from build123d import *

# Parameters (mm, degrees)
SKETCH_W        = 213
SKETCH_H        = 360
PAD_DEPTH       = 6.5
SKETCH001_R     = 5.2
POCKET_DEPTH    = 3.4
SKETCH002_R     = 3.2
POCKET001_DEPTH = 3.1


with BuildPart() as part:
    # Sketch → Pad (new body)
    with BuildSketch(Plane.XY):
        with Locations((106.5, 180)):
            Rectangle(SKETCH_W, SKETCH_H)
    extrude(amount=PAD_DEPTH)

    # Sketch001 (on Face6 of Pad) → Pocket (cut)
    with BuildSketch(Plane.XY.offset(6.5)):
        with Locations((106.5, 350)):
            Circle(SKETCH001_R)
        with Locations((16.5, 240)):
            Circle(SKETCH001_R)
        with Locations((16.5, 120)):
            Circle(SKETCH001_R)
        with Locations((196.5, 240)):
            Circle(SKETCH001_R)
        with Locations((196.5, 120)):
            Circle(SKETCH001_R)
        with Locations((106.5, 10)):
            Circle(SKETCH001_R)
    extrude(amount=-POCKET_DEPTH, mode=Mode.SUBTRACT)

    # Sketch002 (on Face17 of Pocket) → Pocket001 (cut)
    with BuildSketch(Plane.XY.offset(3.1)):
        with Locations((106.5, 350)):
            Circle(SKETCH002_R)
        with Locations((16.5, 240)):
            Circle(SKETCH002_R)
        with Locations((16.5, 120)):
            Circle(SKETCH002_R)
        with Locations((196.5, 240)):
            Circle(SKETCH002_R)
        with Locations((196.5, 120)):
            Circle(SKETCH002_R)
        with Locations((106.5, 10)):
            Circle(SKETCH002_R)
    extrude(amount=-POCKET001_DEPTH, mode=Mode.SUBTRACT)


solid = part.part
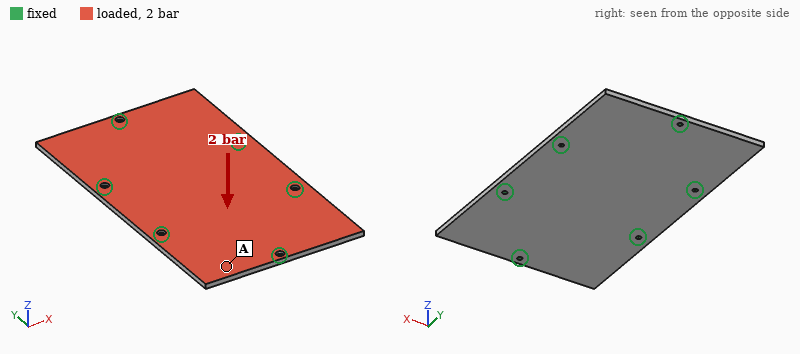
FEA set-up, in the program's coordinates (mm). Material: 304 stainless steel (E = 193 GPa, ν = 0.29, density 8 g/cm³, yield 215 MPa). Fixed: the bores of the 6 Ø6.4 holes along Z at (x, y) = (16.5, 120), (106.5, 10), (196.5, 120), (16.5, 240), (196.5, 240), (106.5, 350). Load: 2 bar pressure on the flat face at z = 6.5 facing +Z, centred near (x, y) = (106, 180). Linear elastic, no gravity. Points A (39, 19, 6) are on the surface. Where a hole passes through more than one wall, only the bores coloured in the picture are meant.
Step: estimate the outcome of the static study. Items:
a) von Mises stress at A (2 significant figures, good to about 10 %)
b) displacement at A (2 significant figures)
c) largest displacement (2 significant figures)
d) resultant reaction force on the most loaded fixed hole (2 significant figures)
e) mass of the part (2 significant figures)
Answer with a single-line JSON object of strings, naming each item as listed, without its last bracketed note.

{"von Mises stress at A": "35 MPa", "displacement at A": "0.14 mm", "largest displacement": "0.23 mm", "resultant reaction force on the most loaded fixed hole": "4.0 kN", "mass of the part": "4.0 kg"}
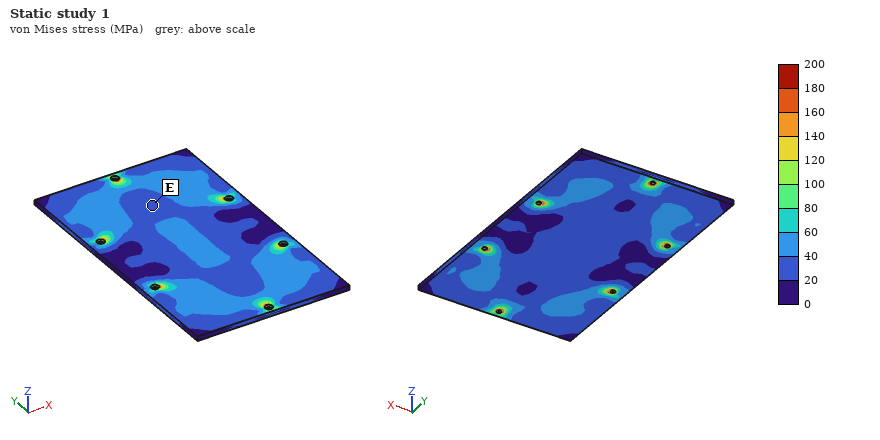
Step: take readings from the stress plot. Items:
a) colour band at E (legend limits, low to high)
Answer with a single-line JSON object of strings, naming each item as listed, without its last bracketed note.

{"colour band at E": "20 to 40 MPa"}
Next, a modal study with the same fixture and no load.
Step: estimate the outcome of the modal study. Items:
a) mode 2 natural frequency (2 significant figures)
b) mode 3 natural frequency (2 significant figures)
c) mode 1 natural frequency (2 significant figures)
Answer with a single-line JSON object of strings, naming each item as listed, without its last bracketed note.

{"mode 2 natural frequency": "660 Hz", "mode 3 natural frequency": "700 Hz", "mode 1 natural frequency": "650 Hz"}
